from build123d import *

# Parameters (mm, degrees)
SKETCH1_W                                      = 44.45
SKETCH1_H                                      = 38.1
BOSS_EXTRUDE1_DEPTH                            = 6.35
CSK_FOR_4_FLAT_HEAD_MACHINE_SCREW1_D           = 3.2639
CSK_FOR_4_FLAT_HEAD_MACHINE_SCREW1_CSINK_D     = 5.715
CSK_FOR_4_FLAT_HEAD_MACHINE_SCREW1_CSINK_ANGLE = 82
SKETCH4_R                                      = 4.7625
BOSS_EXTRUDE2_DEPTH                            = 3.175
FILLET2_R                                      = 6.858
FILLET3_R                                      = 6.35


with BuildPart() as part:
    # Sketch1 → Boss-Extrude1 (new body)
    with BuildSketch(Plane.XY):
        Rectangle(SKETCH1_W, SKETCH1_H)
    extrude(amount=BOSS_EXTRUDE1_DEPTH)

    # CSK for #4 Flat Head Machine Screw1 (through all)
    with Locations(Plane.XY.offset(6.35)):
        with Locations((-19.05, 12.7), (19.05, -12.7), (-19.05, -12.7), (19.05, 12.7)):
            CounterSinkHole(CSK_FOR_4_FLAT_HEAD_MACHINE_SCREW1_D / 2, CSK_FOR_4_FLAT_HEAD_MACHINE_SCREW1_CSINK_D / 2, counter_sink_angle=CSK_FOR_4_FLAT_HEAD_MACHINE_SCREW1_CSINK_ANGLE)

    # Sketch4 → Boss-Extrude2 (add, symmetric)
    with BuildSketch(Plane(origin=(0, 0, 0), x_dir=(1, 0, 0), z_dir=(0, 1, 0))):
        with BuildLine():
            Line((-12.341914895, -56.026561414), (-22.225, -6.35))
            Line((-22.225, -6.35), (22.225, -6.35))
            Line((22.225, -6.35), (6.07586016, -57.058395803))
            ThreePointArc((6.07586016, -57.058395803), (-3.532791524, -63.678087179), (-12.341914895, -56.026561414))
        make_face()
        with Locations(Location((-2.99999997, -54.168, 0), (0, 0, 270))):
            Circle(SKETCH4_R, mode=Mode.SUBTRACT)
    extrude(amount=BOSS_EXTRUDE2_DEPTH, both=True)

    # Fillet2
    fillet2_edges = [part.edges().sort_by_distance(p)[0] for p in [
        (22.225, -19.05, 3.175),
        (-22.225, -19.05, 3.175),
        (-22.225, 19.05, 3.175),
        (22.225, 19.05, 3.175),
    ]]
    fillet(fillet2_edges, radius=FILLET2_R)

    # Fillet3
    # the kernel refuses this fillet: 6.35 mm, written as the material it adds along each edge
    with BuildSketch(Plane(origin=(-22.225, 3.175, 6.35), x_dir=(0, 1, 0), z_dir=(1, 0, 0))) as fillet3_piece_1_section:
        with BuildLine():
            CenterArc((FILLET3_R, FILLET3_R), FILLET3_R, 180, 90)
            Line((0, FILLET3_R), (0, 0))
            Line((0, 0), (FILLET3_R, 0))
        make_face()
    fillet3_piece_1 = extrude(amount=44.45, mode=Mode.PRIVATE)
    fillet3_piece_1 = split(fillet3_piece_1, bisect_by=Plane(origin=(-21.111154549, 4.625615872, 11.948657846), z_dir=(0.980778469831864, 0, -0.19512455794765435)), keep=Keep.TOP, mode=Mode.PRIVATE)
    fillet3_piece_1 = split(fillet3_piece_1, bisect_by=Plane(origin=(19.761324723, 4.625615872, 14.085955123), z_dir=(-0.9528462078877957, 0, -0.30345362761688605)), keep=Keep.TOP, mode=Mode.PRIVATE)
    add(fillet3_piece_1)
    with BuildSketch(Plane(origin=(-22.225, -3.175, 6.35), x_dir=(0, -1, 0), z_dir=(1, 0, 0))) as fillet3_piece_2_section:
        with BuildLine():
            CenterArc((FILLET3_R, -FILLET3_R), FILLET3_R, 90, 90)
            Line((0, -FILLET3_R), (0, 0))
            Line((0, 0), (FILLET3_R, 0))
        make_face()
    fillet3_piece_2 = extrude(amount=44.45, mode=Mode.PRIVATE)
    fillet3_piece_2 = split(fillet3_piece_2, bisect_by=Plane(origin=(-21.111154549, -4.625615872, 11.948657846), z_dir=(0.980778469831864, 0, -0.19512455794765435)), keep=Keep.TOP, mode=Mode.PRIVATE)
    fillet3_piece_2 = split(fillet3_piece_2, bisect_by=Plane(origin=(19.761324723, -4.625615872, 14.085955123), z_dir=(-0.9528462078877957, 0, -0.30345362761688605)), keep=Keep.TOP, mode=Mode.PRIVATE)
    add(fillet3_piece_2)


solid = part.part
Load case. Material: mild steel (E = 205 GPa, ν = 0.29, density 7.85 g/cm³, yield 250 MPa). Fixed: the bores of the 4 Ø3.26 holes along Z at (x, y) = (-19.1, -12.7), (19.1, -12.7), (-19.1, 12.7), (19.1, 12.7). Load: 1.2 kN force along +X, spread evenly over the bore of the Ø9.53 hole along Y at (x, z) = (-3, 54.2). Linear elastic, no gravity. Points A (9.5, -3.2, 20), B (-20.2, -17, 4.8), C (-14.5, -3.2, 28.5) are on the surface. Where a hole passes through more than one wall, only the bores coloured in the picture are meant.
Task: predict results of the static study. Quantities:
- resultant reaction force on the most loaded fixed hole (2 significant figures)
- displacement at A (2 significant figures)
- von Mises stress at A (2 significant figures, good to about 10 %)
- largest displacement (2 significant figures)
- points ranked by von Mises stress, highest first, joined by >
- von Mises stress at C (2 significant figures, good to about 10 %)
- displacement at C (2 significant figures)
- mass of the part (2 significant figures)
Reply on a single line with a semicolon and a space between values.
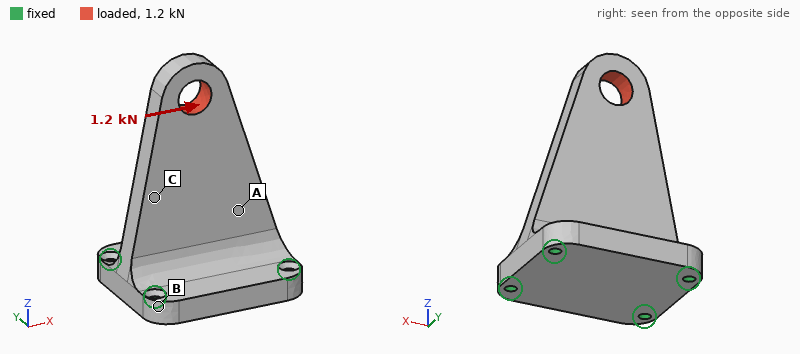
990 N; 4.4 µm; 18 MPa; 25 µm; C > A > B; 23 MPa; 7.8 µm; 170 g
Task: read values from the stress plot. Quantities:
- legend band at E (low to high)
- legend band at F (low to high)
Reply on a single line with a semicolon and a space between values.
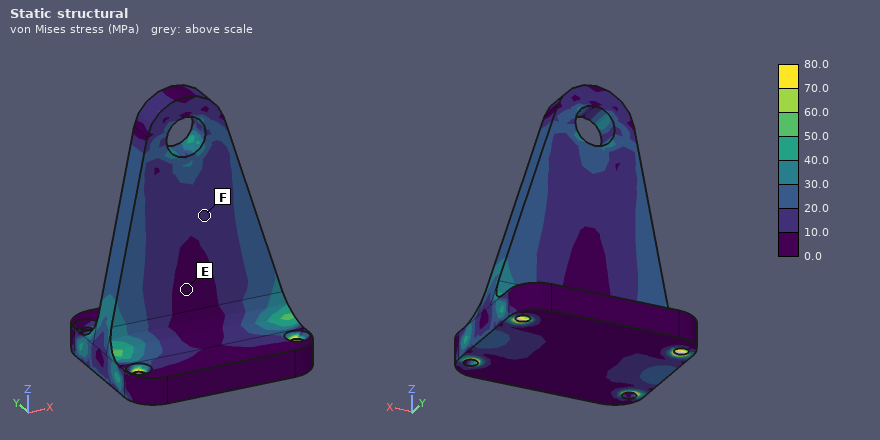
0.0 to 10.0 MPa; 10.0 to 20.0 MPa
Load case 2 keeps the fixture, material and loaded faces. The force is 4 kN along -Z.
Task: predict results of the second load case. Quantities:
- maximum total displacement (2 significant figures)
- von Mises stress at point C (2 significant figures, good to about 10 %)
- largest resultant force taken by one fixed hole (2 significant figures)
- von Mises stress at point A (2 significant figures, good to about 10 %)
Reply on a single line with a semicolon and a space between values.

12 µm; 25 MPa; 1.3 kN; 14 MPa
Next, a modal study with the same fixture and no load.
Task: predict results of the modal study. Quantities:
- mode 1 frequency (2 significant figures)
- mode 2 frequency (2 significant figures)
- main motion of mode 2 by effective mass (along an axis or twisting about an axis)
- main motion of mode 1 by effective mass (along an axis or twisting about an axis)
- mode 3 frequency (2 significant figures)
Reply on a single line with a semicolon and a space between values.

2500 Hz; 8100 Hz; along X; along Y; 9800 Hz
